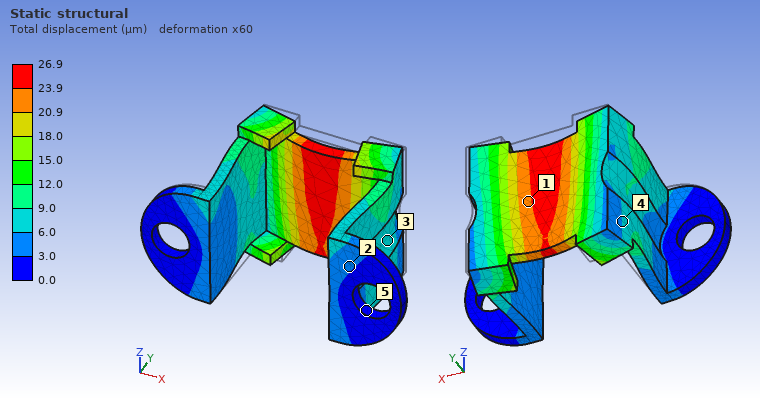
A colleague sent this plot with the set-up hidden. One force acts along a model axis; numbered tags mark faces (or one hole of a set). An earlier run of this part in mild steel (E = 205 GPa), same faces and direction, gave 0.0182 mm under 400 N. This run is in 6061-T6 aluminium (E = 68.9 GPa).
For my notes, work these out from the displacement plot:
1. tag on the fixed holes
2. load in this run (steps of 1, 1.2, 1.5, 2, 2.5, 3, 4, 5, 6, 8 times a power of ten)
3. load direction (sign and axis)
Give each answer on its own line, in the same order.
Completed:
5
200 N
-Y
